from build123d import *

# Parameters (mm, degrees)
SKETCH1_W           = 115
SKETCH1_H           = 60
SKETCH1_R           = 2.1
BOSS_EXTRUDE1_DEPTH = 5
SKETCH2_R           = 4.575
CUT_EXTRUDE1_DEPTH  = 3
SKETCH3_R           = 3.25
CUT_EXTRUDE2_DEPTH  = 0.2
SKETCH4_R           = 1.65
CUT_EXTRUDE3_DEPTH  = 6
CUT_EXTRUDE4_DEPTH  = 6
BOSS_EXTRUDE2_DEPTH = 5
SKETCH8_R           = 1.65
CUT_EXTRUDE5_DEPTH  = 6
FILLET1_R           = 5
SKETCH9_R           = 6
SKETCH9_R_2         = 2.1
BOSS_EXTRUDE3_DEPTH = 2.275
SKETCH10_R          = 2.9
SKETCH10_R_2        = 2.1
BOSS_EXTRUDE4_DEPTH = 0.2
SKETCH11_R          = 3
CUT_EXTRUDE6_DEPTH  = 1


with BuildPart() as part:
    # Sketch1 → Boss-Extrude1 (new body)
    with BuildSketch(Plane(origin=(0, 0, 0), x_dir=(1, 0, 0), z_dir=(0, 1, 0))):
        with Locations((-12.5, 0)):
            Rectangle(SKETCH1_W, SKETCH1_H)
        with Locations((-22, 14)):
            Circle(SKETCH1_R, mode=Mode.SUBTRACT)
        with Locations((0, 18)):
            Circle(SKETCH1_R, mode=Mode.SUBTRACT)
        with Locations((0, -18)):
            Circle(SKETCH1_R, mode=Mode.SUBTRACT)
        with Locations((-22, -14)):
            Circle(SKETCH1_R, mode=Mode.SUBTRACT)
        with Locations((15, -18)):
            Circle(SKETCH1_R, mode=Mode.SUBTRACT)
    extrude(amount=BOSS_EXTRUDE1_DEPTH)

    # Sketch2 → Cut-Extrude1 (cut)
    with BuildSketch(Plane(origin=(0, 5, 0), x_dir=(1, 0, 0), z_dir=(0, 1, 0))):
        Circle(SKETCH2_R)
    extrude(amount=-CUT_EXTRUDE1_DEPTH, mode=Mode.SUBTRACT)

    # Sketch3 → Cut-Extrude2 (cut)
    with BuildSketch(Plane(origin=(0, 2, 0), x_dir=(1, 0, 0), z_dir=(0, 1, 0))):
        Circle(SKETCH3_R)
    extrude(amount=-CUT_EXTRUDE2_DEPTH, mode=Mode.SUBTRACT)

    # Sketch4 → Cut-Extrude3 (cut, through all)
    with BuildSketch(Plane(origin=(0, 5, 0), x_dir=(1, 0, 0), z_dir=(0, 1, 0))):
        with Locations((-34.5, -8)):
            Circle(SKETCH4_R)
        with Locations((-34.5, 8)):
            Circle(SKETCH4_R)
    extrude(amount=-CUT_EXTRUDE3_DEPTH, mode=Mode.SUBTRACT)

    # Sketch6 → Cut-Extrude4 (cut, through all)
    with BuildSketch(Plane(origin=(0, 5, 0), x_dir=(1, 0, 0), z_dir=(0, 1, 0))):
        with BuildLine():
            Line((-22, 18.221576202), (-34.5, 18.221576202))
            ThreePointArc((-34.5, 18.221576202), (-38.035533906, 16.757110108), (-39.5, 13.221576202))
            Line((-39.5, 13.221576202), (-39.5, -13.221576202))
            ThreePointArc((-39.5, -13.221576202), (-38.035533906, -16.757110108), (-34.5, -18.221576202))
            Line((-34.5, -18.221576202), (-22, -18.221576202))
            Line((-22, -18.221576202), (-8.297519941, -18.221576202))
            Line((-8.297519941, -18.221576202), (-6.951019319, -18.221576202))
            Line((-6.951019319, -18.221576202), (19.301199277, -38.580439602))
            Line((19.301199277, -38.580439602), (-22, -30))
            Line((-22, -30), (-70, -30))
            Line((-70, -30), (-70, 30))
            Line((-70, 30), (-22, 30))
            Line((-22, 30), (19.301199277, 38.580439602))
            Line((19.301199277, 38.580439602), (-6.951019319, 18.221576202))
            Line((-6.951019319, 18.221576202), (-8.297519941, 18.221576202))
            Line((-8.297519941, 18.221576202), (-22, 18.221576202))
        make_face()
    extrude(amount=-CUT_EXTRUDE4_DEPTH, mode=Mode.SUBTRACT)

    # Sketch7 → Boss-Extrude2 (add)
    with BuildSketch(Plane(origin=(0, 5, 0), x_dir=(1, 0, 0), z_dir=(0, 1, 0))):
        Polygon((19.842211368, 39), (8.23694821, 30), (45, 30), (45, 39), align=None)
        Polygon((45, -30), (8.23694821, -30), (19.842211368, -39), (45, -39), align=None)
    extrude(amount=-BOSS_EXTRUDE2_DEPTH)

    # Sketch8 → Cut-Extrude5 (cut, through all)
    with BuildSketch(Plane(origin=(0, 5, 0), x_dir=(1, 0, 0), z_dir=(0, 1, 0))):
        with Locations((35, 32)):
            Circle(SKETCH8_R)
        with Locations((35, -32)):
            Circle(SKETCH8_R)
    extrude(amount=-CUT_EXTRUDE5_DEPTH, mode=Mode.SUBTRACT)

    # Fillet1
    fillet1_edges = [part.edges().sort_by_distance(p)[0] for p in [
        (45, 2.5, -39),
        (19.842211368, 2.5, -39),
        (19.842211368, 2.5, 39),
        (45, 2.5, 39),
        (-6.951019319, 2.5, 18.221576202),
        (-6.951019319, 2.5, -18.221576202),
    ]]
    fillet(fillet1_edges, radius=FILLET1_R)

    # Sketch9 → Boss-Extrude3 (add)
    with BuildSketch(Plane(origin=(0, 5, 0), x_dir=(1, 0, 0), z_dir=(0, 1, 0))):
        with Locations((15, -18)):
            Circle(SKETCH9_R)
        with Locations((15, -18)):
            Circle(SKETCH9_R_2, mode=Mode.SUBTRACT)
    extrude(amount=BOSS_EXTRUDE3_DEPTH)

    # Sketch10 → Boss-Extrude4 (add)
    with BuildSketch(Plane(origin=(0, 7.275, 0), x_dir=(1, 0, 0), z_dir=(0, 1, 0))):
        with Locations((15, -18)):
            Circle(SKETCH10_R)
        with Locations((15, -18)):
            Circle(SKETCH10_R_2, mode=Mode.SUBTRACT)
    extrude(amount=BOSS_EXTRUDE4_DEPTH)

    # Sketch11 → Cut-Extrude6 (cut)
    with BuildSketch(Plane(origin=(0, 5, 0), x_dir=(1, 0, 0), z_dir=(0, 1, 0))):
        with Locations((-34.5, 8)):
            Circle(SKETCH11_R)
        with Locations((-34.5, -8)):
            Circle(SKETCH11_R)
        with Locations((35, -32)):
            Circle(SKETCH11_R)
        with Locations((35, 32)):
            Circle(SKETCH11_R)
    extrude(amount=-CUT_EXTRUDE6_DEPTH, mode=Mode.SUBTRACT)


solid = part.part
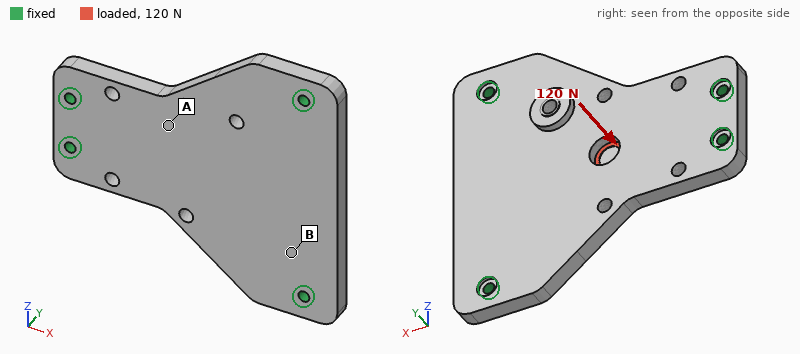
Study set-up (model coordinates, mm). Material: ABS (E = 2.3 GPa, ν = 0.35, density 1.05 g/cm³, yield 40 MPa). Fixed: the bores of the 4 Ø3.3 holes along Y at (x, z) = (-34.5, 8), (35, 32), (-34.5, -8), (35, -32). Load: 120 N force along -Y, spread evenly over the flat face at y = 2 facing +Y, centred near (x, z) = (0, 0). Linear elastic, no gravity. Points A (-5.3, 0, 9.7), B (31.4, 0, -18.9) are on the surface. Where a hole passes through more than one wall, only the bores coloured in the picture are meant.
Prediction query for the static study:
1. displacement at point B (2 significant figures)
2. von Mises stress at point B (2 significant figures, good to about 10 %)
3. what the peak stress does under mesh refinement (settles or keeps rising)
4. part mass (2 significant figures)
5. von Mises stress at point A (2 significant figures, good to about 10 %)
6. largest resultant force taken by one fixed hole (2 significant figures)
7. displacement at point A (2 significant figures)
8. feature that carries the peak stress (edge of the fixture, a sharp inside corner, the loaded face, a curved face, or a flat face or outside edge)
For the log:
0.073 mm
1.6 MPa
keeps rising
24 g
5.1 MPa
33 N
0.31 mm
edge of the fixture
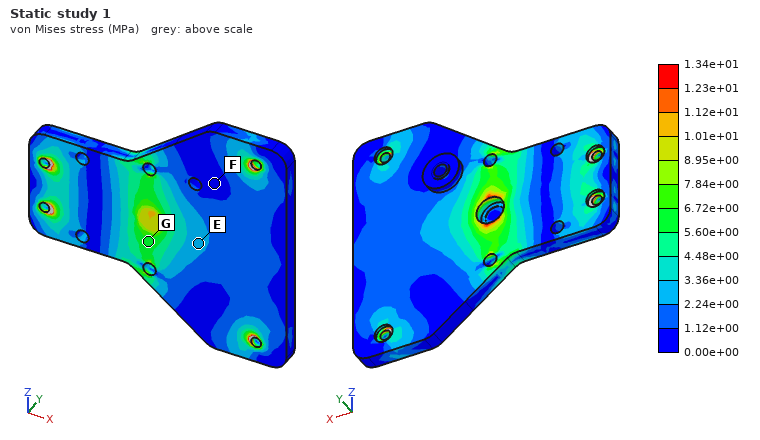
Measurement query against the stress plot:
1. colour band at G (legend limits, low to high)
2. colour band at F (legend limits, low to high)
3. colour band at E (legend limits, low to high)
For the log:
5.60e+00 to 6.72e+00 MPa
0.00e+00 to 1.12e+00 MPa
2.24e+00 to 3.36e+00 MPa
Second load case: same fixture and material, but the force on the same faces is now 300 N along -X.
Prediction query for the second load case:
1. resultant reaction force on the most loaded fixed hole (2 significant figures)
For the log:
86 N
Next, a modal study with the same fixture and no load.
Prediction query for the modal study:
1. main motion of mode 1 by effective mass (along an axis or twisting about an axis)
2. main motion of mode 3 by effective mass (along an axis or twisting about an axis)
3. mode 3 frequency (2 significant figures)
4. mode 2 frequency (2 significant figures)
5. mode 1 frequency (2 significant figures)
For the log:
along Y
twisting about X
1800 Hz
1700 Hz
1100 Hz
